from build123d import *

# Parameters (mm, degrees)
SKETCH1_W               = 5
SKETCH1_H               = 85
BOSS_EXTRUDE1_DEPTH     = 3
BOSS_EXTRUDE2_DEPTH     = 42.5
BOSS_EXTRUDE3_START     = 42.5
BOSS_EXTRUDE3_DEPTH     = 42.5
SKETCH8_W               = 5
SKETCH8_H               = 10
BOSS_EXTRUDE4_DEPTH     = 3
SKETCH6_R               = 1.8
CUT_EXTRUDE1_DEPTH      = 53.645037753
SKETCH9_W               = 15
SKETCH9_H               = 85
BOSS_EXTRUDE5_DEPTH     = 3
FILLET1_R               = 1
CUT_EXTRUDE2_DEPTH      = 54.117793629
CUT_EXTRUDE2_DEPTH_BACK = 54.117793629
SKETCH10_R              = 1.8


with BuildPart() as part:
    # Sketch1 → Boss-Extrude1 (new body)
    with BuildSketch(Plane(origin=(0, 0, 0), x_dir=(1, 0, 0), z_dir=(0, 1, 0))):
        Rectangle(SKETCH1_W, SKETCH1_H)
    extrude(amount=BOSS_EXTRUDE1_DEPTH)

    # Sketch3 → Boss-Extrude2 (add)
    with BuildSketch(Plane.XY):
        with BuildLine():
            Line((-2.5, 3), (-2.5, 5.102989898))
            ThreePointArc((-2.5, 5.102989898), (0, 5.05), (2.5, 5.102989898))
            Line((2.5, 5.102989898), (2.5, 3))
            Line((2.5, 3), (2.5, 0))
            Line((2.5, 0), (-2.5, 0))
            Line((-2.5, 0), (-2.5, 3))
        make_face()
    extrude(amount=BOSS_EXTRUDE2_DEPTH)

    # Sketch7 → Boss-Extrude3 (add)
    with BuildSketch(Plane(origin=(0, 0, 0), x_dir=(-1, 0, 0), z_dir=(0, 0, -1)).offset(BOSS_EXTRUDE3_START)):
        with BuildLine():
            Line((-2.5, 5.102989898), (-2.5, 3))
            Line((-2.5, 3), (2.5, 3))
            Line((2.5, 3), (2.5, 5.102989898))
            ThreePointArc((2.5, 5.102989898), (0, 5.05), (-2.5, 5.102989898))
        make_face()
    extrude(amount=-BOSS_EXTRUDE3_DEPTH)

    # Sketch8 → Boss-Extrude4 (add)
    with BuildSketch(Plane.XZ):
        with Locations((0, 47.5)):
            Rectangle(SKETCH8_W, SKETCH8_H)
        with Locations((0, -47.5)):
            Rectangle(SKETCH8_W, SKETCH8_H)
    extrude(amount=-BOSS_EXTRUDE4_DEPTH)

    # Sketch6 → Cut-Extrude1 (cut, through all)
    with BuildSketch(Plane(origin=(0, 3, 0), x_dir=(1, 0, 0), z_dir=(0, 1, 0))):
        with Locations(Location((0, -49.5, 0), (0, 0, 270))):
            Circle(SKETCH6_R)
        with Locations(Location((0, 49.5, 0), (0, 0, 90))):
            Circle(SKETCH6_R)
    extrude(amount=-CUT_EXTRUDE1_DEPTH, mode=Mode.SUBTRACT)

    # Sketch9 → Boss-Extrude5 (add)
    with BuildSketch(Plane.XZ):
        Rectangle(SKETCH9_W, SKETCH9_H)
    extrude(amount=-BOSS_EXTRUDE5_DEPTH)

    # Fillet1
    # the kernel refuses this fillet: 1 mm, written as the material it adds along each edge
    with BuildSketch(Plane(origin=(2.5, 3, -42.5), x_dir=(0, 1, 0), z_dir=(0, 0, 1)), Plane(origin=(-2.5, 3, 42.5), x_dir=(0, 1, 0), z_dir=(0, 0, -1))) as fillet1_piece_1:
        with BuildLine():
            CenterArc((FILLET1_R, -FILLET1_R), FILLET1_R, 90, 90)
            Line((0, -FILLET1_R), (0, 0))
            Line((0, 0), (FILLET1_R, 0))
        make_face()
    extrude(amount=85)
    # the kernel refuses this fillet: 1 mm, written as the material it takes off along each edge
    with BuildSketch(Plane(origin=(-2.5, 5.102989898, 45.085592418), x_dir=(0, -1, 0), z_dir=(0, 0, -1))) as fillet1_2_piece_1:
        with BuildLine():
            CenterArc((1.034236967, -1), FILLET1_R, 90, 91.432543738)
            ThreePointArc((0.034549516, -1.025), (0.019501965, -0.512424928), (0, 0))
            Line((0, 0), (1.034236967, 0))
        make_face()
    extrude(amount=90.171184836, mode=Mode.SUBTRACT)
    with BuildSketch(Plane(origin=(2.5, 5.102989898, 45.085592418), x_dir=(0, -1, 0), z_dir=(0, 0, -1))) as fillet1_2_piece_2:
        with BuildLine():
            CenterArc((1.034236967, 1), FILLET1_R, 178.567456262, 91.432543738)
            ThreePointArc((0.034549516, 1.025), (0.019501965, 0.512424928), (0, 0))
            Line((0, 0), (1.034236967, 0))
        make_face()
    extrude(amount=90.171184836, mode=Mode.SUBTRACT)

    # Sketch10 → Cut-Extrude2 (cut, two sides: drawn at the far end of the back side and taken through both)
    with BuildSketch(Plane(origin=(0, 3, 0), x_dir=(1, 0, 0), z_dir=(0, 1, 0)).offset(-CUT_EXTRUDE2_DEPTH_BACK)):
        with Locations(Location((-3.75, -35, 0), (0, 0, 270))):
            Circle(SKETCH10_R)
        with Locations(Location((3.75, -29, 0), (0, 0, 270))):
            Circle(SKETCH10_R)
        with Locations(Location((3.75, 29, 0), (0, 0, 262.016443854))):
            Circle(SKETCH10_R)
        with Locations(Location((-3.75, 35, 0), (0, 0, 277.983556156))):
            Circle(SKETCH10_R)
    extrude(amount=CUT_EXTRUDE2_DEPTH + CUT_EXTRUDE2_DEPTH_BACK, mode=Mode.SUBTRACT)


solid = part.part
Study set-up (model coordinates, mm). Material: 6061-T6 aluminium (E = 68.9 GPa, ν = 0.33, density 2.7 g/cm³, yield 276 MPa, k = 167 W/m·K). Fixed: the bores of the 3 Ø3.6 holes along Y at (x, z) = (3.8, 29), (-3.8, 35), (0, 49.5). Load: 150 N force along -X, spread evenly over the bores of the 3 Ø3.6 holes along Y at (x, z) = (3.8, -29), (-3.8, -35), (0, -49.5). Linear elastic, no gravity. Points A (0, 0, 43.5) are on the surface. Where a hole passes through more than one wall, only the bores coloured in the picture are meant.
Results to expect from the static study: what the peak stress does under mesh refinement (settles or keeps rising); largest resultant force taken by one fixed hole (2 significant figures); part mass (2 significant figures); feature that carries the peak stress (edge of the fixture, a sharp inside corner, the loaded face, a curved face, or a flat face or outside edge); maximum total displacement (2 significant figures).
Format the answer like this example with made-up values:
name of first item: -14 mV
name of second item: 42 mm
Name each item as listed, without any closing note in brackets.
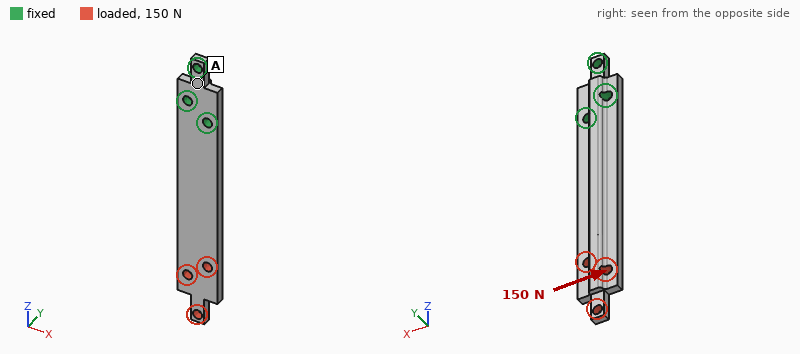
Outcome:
what the peak stress does under mesh refinement: keeps rising
largest resultant force taken by one fixed hole: 950 N
part mass: 13 g
feature that carries the peak stress: edge of the fixture
maximum total displacement: 0.38 mm
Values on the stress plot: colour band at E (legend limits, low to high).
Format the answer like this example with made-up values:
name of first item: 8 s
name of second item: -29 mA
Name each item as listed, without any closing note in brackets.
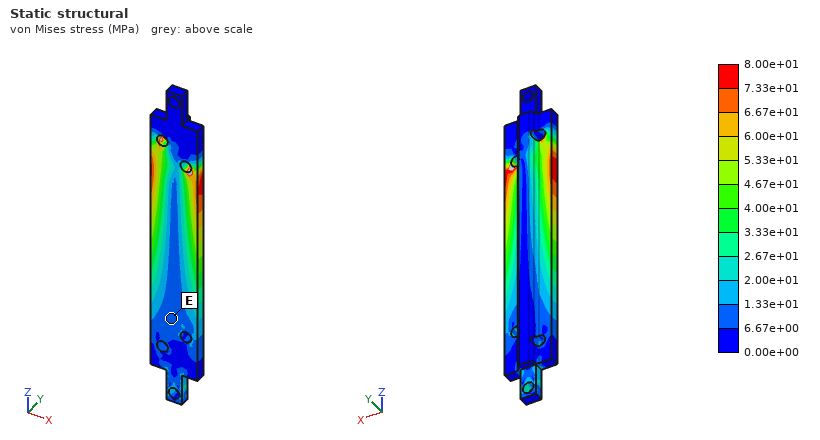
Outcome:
colour band at E: 6.67e+00 to 1.33e+01 MPa
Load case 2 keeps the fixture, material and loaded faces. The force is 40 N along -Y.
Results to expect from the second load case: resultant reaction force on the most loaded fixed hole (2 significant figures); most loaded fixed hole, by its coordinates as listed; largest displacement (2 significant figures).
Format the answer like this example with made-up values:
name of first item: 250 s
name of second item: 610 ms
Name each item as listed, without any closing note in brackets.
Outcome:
resultant reaction force on the most loaded fixed hole: 160 N
most loaded fixed hole, by its coordinates as listed: (3.8, 29)
largest displacement: 0.88 mm
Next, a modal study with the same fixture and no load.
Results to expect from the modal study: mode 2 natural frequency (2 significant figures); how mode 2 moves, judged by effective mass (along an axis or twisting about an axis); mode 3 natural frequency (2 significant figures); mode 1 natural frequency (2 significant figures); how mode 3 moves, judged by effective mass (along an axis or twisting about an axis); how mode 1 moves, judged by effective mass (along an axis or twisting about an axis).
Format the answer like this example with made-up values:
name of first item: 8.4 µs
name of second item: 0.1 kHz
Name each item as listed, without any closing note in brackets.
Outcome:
mode 2 natural frequency: 1900 Hz
how mode 2 moves, judged by effective mass: along X
mode 3 natural frequency: 3800 Hz
mode 1 natural frequency: 660 Hz
how mode 3 moves, judged by effective mass: along Y
how mode 1 moves, judged by effective mass: along Y
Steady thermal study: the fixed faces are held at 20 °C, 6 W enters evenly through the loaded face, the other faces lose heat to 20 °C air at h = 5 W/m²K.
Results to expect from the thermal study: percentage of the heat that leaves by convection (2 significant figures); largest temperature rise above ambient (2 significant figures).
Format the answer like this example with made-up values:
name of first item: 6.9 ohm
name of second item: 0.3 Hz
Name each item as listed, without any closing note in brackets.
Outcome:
percentage of the heat that leaves by convection: 5.7 %
largest temperature rise above ambient: 50 K
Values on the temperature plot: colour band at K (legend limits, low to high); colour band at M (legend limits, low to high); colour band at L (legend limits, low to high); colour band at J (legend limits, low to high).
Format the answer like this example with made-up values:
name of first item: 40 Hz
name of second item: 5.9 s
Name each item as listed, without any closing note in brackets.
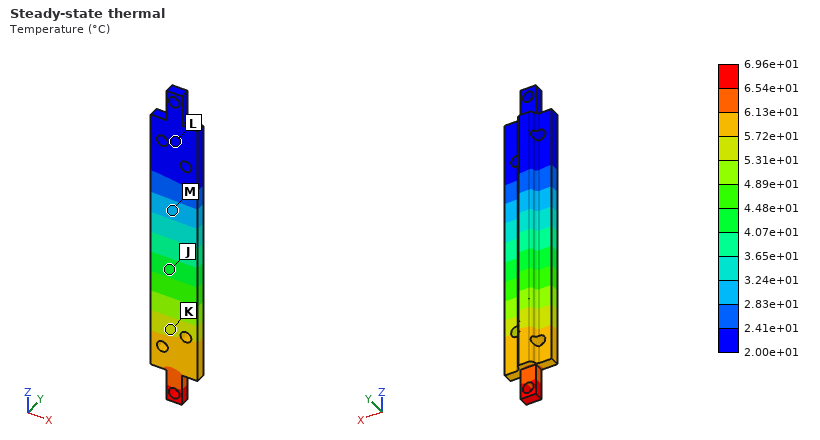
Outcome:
colour band at K: 5.31e+01 to 5.72e+01 °C
colour band at M: 2.83e+01 to 3.24e+01 °C
colour band at L: 2.00e+01 to 2.41e+01 °C
colour band at J: 4.07e+01 to 4.48e+01 °C
